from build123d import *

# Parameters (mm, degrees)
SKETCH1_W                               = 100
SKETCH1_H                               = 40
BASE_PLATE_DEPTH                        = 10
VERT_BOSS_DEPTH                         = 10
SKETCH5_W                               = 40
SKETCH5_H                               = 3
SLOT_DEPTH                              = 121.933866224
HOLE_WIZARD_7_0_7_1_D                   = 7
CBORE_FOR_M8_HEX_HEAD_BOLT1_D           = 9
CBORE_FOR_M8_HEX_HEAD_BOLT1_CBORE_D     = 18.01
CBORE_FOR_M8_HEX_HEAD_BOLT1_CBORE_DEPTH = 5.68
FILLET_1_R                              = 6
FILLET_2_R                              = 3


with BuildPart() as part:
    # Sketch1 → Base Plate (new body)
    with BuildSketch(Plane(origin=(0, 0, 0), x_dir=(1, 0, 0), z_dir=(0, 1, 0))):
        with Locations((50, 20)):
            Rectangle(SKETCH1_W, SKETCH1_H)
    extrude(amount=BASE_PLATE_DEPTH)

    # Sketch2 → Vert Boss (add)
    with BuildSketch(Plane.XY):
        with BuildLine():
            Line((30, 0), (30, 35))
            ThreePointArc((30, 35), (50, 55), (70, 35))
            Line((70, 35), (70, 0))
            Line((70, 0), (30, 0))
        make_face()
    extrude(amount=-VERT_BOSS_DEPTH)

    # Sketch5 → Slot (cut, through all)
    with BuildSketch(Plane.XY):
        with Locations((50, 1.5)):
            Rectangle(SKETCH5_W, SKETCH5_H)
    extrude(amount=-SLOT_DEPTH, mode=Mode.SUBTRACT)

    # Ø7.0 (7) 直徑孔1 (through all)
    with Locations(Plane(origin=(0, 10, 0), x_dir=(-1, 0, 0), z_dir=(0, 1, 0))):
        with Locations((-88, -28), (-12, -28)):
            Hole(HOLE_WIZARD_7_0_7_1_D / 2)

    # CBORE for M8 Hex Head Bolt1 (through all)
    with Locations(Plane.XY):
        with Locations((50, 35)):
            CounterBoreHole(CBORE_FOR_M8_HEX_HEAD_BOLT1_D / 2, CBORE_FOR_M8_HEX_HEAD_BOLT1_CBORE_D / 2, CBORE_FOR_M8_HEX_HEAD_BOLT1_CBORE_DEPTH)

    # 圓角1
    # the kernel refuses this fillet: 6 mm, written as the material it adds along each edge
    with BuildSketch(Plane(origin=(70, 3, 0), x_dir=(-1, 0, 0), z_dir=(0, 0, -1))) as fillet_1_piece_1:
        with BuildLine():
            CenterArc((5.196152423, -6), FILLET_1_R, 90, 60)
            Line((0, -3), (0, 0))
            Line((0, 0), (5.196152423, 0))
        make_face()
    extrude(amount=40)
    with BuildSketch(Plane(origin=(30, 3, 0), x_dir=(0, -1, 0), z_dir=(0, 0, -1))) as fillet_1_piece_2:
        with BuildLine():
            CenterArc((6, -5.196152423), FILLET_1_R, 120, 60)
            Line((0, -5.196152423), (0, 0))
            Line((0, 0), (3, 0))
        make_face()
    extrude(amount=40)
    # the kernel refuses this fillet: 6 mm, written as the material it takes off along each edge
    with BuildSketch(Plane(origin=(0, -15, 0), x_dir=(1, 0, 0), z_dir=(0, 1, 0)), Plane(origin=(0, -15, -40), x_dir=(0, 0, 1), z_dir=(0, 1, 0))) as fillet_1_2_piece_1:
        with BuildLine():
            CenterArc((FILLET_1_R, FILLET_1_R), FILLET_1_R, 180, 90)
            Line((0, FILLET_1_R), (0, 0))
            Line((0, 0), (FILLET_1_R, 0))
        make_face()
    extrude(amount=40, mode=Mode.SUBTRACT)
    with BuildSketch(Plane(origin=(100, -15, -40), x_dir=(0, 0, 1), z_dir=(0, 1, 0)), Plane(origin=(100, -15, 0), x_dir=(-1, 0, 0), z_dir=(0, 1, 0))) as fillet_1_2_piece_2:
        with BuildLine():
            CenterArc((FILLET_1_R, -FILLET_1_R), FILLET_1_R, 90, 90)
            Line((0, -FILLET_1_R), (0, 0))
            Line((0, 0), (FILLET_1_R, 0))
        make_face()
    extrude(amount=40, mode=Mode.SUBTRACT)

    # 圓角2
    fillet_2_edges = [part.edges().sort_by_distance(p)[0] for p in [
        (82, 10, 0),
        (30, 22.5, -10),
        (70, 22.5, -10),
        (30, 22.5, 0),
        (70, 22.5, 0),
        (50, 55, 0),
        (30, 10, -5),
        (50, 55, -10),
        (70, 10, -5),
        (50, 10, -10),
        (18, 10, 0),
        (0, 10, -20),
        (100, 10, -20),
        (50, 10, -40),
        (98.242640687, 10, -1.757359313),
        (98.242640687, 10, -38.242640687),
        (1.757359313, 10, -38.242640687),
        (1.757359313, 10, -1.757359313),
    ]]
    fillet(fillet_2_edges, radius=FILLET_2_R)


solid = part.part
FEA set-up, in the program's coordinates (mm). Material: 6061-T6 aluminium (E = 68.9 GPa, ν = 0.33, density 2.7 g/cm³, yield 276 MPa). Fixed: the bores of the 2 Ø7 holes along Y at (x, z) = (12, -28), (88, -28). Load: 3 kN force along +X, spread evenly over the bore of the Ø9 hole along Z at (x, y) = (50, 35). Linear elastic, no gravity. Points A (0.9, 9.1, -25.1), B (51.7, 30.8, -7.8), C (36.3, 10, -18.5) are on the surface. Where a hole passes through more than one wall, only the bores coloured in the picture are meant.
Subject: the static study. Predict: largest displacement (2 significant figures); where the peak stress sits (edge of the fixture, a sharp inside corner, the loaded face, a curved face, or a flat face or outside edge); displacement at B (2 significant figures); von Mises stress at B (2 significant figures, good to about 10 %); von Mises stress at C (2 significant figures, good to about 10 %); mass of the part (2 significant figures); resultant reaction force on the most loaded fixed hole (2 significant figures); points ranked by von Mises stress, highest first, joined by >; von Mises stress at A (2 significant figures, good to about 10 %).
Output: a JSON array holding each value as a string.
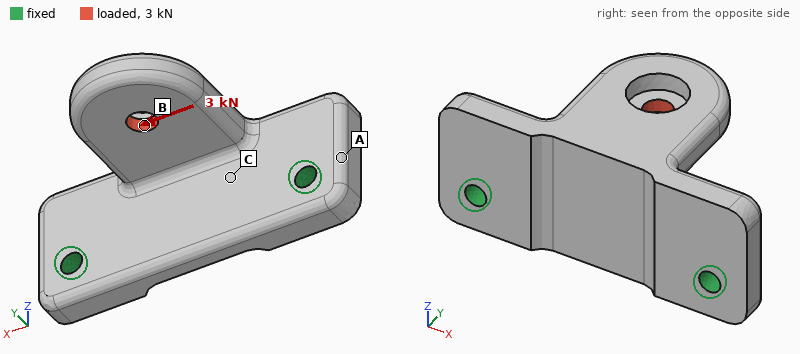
["0.12 mm", "a curved face", "0.064 mm", "55 MPa", "35 MPa", "130 g", "2.2 kN", "B > C > A", "14 MPa"]
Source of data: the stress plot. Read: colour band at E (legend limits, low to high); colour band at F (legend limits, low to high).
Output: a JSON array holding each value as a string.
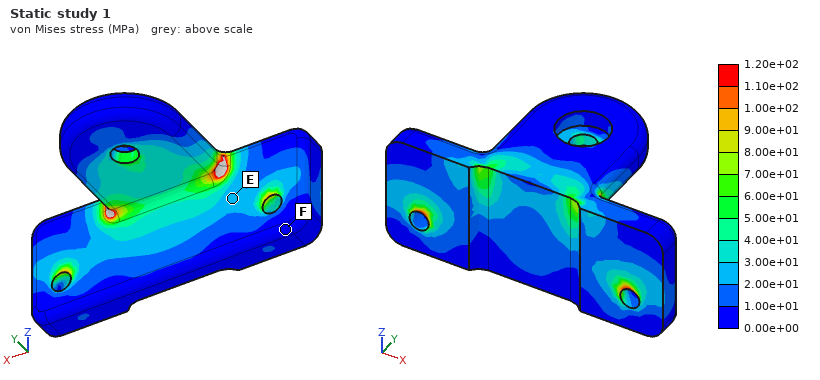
["2.00e+01 to 3.00e+01 MPa", "0.00e+00 to 1.00e+01 MPa"]
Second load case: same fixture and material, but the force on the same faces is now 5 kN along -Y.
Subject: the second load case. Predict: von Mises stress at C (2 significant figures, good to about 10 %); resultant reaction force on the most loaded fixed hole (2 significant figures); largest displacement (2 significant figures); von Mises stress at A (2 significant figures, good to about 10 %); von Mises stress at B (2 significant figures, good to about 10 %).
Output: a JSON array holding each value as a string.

["28 MPa", "2.7 kN", "0.19 mm", "33 MPa", "42 MPa"]
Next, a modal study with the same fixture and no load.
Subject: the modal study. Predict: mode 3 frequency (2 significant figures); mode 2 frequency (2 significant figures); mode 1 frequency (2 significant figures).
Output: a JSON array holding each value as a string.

["5100 Hz", "5000 Hz", "2300 Hz"]
